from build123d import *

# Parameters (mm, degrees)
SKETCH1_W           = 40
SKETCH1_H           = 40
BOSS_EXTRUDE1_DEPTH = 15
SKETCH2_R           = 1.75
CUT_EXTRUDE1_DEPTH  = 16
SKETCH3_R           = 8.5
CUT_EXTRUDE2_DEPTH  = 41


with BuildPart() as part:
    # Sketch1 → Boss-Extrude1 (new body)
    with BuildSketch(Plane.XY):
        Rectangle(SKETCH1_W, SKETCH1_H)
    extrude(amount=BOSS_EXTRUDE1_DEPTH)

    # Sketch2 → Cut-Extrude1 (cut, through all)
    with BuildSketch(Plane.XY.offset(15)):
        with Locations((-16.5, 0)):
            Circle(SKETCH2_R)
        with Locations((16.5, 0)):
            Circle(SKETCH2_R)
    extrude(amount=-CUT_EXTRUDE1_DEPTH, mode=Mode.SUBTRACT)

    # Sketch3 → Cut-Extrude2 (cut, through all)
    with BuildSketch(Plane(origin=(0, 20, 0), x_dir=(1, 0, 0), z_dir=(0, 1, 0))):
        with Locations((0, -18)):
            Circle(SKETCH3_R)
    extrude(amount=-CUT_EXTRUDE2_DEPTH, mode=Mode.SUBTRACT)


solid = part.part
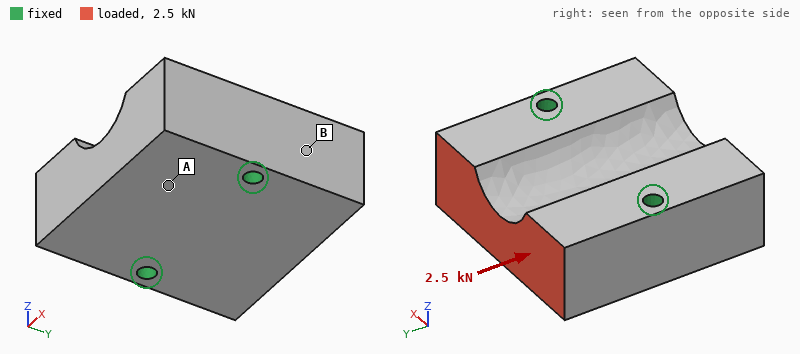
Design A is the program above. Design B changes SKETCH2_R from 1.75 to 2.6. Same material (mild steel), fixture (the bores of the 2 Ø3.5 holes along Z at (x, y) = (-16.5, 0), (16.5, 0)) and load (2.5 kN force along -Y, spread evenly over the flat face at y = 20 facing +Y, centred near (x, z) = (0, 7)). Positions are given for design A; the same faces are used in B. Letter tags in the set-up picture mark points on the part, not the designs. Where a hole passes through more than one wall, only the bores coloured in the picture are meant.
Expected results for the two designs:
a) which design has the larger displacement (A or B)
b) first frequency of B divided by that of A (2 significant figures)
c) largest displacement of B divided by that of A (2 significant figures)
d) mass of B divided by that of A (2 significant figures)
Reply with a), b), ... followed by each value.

a) A
b) 1.1
c) 0.90
d) 0.98
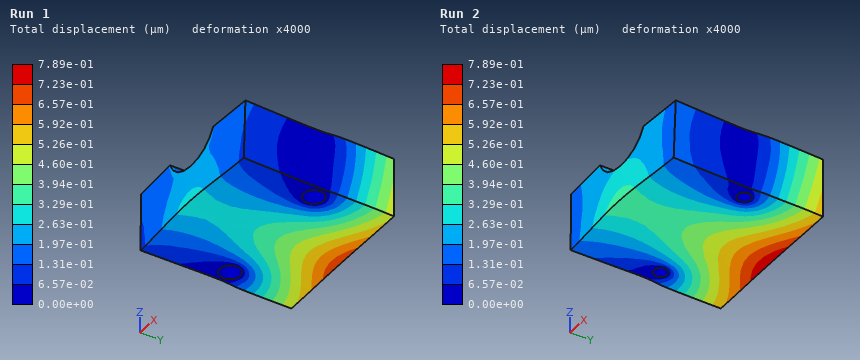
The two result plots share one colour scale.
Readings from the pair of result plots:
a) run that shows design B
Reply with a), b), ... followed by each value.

a) Run 1
